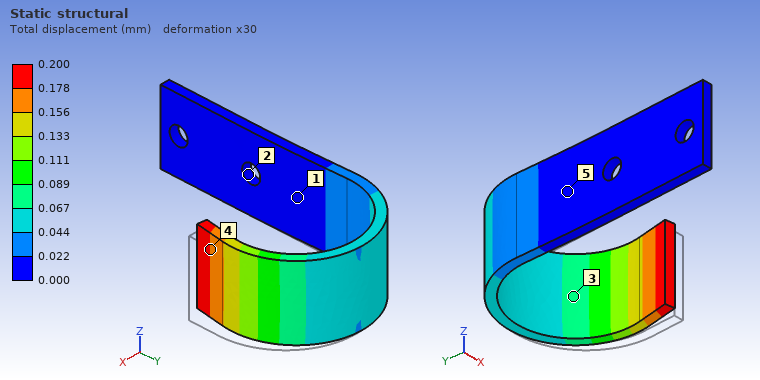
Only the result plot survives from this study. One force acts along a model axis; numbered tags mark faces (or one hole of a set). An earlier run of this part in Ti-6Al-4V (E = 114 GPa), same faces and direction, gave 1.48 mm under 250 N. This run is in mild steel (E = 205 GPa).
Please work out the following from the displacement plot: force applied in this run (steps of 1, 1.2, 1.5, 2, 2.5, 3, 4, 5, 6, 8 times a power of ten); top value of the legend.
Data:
60 N
0.200 mm
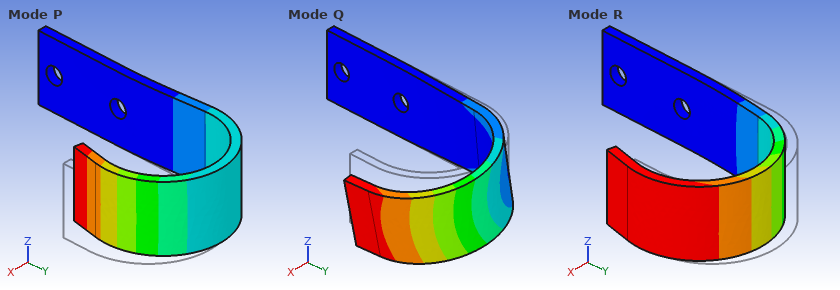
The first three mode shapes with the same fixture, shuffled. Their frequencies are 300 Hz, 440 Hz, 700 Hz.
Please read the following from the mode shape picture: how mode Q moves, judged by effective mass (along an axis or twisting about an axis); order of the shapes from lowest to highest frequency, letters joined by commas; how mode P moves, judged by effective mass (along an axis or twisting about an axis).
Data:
along Z
R, Q, P
along X
